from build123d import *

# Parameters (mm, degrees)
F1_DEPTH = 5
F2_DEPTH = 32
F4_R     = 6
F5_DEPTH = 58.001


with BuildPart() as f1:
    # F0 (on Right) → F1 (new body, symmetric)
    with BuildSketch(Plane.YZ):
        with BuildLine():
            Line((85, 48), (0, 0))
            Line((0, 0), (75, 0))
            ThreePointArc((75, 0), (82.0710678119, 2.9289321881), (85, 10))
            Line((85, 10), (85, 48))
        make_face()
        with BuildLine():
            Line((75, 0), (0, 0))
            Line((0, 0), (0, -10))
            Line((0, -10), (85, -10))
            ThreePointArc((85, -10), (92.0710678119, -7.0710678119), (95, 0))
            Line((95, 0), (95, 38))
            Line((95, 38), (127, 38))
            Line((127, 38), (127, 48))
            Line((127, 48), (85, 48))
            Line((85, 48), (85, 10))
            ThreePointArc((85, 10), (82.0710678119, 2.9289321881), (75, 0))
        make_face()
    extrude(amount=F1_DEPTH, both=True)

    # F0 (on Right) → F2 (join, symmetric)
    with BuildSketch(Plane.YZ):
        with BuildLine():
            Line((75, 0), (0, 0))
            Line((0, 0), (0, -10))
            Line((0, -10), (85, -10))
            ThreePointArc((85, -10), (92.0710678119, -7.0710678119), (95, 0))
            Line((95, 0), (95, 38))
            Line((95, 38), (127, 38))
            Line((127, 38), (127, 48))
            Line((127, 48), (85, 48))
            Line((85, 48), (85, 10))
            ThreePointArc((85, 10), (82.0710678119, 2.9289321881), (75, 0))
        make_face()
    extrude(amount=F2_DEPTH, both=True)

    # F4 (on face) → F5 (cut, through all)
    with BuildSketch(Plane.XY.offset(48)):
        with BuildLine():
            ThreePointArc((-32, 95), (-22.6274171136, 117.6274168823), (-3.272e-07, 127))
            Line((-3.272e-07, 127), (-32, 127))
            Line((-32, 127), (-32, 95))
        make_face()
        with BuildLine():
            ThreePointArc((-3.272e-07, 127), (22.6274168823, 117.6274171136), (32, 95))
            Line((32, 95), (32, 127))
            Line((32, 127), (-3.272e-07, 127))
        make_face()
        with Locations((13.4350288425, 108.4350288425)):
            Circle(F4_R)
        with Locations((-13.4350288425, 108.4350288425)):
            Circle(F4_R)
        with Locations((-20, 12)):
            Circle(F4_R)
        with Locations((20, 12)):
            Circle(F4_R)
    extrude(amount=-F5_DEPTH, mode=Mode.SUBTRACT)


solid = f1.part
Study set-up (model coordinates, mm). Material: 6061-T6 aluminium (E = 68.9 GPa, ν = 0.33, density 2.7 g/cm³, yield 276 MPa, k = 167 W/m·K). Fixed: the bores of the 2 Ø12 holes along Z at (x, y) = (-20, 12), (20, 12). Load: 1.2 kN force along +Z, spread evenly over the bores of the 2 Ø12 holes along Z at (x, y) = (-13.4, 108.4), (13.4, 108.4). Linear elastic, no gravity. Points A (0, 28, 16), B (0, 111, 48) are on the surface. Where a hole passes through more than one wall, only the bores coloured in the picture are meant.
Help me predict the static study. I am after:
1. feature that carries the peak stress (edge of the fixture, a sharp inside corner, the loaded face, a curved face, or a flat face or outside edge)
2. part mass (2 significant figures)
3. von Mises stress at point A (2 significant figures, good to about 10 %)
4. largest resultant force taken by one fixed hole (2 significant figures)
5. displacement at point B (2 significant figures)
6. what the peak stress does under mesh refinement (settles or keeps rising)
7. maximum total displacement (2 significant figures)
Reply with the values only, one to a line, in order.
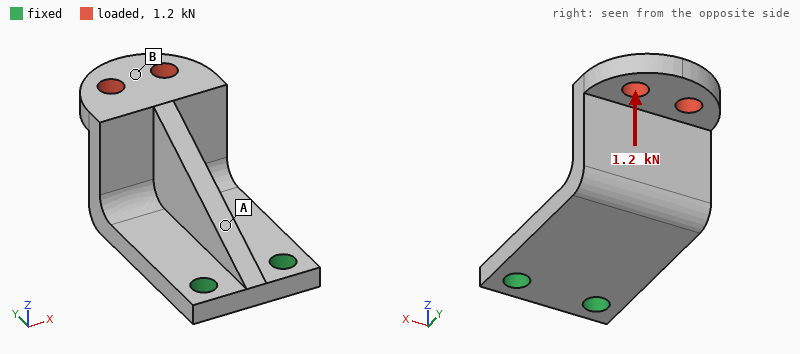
edge of the fixture
330 g
45 MPa
620 N
0.40 mm
keeps rising
0.47 mm
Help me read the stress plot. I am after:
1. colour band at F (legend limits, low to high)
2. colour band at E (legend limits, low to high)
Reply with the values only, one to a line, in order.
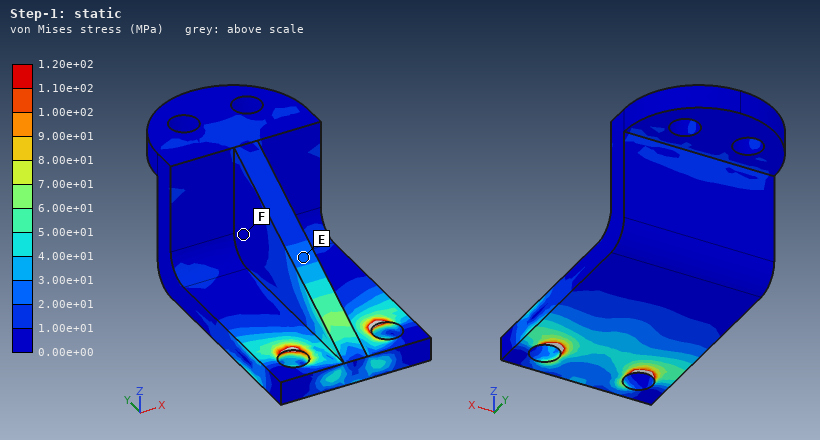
0.00e+00 to 1.00e+01 MPa
2.00e+01 to 3.00e+01 MPa
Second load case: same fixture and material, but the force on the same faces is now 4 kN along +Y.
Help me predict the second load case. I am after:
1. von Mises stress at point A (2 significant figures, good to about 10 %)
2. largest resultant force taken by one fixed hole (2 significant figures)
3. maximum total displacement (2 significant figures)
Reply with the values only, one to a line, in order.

99 MPa
2.0 kN
0.83 mm
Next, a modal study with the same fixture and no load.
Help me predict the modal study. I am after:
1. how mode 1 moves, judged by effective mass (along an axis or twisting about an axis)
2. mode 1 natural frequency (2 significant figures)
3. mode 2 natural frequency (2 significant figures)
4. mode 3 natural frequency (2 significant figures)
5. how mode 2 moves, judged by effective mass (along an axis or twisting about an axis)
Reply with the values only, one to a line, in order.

along Z
780 Hz
1200 Hz
3600 Hz
along X
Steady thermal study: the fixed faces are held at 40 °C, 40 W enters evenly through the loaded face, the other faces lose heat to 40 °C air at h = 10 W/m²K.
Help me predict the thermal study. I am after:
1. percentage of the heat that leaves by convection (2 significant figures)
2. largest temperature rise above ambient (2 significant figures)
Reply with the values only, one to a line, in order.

11 %
37 K
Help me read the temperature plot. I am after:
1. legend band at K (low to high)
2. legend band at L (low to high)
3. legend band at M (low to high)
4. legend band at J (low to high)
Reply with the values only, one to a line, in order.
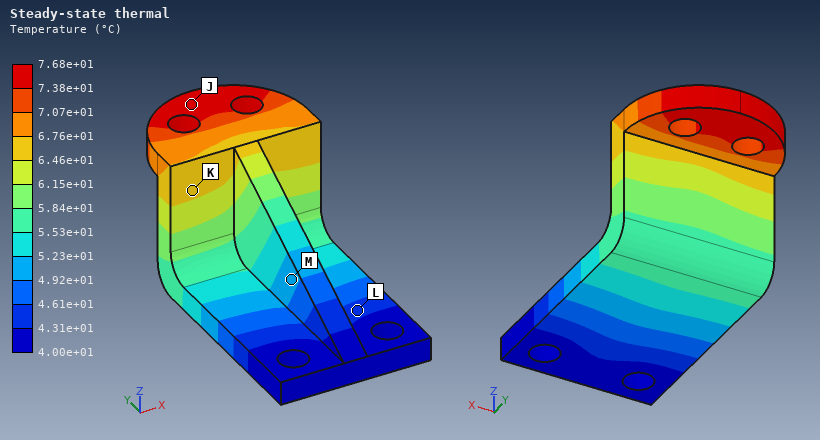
6.46e+01 to 6.76e+01 °C
4.31e+01 to 4.61e+01 °C
4.92e+01 to 5.23e+01 °C
7.38e+01 to 7.68e+01 °C
